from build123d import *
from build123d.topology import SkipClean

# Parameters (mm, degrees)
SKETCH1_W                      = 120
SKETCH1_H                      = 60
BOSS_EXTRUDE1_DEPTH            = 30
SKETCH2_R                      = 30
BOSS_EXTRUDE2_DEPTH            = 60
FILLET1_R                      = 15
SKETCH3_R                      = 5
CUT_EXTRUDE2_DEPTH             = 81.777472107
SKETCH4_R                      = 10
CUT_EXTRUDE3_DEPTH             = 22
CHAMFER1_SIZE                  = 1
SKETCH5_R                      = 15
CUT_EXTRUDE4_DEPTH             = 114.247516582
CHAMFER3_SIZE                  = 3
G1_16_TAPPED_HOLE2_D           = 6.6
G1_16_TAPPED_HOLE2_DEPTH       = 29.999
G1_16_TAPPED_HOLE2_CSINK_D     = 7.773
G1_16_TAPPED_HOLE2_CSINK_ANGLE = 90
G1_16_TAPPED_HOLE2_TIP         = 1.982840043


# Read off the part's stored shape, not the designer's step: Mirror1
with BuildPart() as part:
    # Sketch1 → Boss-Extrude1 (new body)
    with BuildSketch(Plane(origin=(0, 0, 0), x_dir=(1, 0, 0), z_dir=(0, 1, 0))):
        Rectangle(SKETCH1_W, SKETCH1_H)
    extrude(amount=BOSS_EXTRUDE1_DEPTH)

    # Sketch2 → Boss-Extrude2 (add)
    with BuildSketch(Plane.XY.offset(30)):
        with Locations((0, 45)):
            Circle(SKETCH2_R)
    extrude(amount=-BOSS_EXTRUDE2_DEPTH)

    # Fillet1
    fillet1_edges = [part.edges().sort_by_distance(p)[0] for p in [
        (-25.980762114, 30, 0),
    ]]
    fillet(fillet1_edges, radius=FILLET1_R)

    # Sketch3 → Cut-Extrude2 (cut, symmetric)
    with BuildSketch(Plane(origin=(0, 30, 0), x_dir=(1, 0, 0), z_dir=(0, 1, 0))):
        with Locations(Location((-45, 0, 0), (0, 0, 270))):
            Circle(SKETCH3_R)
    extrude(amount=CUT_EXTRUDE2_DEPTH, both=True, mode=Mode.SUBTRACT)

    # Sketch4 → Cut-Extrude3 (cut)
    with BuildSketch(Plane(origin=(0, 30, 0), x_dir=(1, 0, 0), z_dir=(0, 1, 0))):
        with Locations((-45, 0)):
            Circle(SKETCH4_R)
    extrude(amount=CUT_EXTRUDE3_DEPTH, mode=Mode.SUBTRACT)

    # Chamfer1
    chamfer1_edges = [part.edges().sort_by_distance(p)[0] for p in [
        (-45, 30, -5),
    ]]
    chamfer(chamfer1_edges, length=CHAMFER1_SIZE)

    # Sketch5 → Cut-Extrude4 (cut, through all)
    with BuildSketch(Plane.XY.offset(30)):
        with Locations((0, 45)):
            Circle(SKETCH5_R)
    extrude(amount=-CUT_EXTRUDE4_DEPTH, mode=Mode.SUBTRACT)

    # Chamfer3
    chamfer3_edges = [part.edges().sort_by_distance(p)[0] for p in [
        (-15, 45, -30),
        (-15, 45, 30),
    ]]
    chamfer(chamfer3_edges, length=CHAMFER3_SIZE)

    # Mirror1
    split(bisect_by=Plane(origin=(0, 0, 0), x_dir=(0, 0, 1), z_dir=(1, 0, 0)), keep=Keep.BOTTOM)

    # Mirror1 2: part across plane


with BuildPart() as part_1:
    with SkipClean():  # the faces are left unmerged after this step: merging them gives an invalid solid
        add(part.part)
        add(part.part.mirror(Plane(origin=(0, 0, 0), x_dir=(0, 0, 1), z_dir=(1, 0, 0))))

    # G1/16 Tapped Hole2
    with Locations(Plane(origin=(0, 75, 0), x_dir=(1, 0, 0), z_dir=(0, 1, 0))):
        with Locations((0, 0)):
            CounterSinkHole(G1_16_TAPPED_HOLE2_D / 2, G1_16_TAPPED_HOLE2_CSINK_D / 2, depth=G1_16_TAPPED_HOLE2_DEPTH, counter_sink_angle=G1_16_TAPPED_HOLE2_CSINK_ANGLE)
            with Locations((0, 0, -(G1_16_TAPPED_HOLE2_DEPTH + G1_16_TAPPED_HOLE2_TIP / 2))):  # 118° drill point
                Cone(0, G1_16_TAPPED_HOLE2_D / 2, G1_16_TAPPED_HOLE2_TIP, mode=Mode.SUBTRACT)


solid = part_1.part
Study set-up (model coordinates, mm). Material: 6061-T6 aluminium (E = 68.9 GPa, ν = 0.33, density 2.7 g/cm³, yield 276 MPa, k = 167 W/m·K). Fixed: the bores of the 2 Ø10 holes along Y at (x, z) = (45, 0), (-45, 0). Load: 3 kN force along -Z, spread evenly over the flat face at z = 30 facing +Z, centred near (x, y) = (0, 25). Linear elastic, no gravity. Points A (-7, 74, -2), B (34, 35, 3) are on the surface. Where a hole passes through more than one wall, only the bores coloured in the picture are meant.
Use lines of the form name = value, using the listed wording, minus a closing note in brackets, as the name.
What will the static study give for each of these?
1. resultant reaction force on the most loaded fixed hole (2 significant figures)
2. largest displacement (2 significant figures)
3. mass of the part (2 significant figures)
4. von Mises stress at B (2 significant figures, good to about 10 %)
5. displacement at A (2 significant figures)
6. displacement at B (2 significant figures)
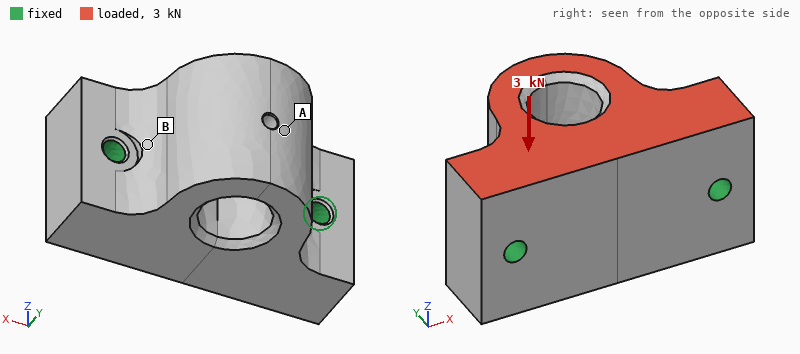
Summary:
resultant reaction force on the most loaded fixed hole = 1.5 kN
largest displacement = 4.7 µm
mass of the part = 840 g
von Mises stress at B = 1.9 MPa
displacement at A = 4.0 µm
displacement at B = 1.4 µm
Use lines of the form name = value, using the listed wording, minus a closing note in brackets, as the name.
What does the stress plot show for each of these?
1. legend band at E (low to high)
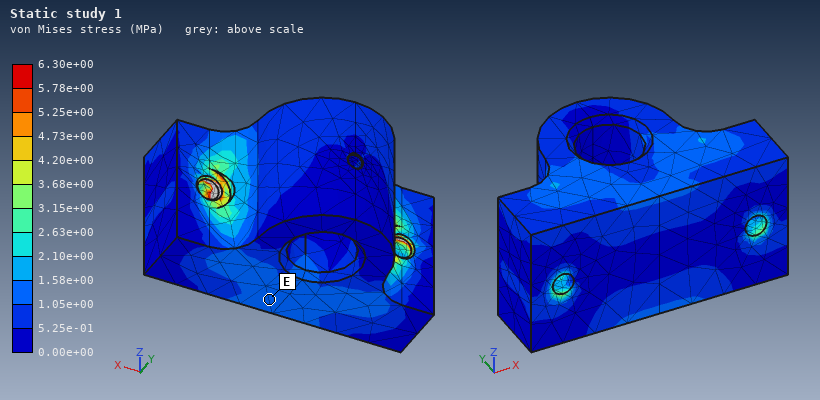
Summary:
legend band at E = 1.05e+00 to 1.58e+00 MPa
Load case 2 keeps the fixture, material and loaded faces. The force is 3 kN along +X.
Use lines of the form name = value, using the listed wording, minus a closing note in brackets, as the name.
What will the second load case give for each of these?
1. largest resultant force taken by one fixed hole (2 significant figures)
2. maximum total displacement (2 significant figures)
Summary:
largest resultant force taken by one fixed hole = 1.8 kN
maximum total displacement = 3.0 µm
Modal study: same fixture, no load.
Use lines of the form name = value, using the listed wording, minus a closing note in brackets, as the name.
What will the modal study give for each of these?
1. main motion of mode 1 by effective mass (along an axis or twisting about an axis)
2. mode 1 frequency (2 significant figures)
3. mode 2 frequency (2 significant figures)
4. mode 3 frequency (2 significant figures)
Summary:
main motion of mode 1 by effective mass = along Z
mode 1 frequency = 5000 Hz
mode 2 frequency = 9000 Hz
mode 3 frequency = 9200 Hz
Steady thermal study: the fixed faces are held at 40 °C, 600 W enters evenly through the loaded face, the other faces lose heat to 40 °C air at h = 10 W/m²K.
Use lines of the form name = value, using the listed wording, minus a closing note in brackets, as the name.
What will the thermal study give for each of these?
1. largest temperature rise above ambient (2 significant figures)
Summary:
largest temperature rise above ambient = 47 K
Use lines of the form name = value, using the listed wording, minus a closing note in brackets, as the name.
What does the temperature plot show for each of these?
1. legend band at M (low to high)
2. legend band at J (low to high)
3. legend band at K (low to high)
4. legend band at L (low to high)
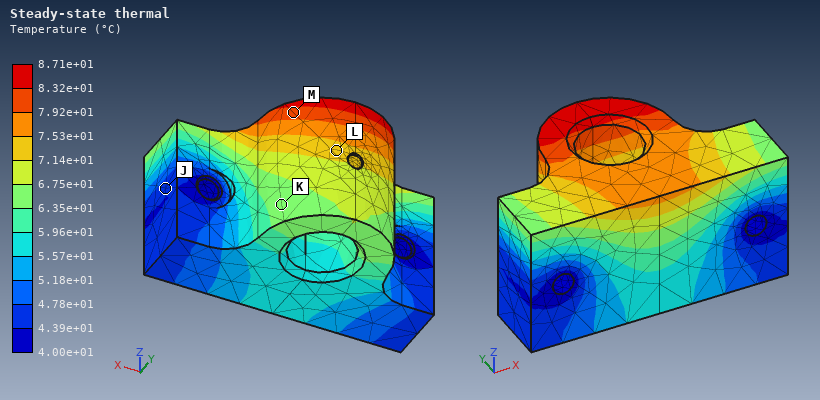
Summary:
legend band at M = 7.92e+01 to 8.32e+01 °C
legend band at J = 4.39e+01 to 4.78e+01 °C
legend band at K = 6.35e+01 to 6.75e+01 °C
legend band at L = 7.14e+01 to 7.53e+01 °C
